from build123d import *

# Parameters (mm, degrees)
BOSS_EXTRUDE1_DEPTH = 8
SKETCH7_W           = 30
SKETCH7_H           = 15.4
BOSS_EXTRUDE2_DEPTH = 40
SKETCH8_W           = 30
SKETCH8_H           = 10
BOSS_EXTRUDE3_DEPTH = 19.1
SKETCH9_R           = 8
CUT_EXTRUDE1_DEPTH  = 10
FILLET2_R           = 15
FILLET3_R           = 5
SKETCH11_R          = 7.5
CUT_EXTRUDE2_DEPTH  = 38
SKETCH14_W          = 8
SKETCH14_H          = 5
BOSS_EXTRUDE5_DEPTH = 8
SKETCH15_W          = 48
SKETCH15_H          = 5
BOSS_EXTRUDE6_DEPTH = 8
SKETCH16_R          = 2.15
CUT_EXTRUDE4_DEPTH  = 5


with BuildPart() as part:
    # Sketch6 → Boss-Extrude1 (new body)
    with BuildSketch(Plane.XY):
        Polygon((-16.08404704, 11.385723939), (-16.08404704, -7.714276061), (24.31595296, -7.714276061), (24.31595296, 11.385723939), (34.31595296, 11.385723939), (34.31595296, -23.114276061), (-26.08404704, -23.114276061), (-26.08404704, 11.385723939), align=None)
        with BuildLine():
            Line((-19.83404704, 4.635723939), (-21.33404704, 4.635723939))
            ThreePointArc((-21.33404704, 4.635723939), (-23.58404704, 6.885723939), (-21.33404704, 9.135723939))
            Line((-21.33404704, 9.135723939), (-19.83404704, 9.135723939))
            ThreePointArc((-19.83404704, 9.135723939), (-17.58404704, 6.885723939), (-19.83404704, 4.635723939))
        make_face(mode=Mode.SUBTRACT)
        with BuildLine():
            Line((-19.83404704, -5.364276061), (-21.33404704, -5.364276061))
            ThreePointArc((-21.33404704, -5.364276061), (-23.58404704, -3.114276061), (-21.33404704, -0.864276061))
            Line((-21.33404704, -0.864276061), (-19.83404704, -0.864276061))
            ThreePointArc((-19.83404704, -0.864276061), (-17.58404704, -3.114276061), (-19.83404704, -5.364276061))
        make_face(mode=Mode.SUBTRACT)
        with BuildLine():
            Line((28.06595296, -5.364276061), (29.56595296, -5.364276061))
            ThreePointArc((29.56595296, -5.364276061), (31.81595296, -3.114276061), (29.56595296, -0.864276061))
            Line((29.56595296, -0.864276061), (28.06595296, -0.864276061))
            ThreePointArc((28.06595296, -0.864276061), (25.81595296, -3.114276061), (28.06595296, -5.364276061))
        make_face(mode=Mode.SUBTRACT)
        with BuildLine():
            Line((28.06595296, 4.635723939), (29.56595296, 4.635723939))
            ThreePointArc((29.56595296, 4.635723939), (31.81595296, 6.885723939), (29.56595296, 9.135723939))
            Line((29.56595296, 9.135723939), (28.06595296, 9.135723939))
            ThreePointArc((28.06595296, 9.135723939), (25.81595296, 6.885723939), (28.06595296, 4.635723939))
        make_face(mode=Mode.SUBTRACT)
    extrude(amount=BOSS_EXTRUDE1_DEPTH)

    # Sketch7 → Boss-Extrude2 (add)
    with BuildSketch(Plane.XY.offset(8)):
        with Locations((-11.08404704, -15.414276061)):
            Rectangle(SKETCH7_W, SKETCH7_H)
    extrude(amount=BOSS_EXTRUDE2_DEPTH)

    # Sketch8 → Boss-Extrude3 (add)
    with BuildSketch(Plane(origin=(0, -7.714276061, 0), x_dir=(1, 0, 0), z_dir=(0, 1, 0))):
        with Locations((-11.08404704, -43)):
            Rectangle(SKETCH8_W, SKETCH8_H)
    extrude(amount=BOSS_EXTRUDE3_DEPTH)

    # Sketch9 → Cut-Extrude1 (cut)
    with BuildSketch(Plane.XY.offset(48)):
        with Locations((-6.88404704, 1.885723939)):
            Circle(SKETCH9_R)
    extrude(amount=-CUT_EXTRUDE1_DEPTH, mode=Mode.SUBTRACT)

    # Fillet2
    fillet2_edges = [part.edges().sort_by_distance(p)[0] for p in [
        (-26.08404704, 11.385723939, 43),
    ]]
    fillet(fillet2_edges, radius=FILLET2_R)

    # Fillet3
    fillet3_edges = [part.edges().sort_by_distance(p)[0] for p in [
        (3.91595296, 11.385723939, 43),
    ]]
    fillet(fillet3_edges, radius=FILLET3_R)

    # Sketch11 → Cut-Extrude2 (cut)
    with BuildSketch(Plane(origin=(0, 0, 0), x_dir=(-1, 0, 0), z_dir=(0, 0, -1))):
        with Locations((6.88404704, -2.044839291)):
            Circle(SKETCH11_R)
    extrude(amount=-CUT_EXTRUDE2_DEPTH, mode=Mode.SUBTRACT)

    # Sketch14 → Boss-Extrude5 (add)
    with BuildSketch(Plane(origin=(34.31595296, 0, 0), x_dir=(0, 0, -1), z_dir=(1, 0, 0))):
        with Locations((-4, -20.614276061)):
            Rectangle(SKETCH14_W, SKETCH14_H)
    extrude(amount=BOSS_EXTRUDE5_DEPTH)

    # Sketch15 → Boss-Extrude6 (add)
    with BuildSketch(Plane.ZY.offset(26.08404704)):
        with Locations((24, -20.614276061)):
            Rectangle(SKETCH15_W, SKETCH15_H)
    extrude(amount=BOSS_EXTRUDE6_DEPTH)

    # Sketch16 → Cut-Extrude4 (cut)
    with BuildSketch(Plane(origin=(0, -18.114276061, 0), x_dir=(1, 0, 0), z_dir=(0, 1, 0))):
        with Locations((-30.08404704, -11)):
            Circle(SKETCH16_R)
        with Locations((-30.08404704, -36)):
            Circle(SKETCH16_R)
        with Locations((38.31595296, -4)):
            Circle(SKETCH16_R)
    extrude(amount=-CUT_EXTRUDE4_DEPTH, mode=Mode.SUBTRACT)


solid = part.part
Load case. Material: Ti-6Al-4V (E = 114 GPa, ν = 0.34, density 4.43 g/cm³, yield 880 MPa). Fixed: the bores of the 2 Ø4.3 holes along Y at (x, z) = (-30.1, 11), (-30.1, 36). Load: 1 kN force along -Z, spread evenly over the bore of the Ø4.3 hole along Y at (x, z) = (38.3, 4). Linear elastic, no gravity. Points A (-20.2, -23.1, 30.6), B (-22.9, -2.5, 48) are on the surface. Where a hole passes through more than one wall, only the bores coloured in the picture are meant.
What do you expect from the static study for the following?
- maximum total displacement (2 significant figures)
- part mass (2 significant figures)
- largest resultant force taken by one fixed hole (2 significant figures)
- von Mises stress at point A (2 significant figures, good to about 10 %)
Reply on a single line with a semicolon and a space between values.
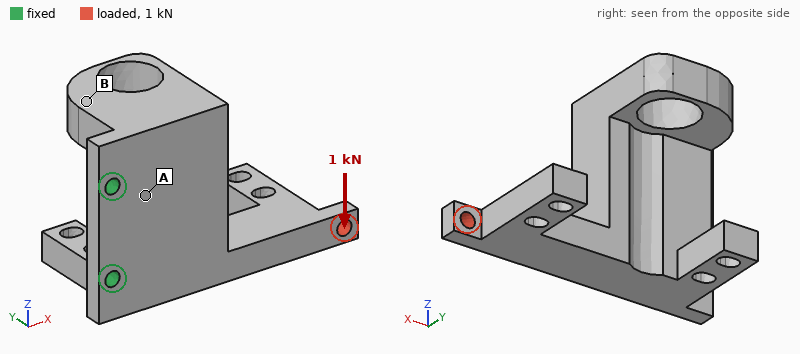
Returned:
0.38 mm; 150 g; 2.6 kN; 32 MPa
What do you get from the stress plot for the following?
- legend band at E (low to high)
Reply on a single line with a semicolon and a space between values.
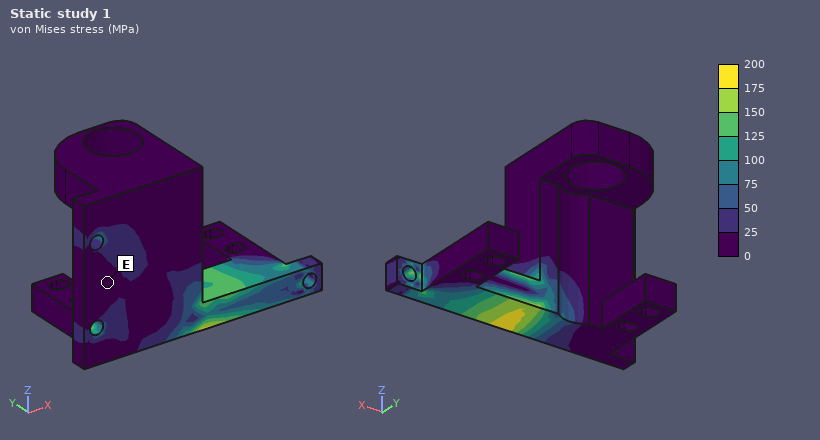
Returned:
0 to 25 MPa
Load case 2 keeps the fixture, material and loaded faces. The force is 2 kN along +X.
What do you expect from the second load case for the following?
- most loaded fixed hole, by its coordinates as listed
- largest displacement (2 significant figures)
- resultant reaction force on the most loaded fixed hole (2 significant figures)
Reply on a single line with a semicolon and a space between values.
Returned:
(-30.1, 11); 64 µm; 2.4 kN
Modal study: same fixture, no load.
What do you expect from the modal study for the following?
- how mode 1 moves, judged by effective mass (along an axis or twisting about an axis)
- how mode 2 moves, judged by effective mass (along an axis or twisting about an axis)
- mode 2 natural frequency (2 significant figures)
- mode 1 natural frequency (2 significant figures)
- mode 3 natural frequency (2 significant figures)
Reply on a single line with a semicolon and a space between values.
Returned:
along Y; along Z; 3200 Hz; 1200 Hz; 4600 Hz
